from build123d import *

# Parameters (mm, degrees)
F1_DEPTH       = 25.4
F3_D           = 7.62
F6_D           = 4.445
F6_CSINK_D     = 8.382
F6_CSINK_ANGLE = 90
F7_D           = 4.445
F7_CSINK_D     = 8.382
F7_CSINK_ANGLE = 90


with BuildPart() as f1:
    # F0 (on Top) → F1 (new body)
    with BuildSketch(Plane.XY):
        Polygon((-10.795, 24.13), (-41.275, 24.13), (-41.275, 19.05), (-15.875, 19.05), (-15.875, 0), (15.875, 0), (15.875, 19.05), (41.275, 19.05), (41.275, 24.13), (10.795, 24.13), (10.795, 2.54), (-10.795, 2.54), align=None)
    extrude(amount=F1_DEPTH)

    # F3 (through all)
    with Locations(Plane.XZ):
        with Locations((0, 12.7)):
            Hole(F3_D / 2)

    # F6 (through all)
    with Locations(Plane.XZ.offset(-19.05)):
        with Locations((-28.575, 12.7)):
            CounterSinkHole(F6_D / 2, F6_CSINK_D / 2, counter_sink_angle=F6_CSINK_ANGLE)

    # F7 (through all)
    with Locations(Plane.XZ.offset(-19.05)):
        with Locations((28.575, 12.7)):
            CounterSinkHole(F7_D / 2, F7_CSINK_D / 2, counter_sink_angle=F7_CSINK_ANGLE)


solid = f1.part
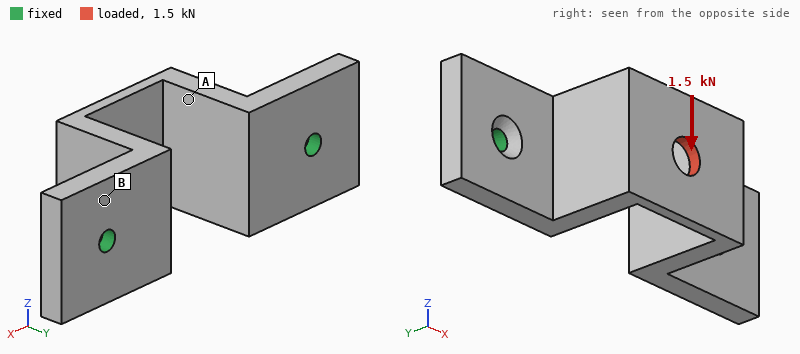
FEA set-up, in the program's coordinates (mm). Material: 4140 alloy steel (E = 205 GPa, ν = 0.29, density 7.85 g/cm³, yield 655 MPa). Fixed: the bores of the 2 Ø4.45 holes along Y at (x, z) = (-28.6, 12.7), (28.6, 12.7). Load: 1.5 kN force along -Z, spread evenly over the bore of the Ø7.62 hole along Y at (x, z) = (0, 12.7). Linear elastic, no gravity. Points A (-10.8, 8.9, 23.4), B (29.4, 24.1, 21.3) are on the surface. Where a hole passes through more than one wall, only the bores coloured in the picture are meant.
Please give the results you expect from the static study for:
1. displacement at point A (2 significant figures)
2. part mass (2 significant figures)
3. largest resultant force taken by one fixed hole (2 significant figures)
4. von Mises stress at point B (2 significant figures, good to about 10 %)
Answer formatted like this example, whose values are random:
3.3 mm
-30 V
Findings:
0.069 mm
110 g
750 N
81 MPa
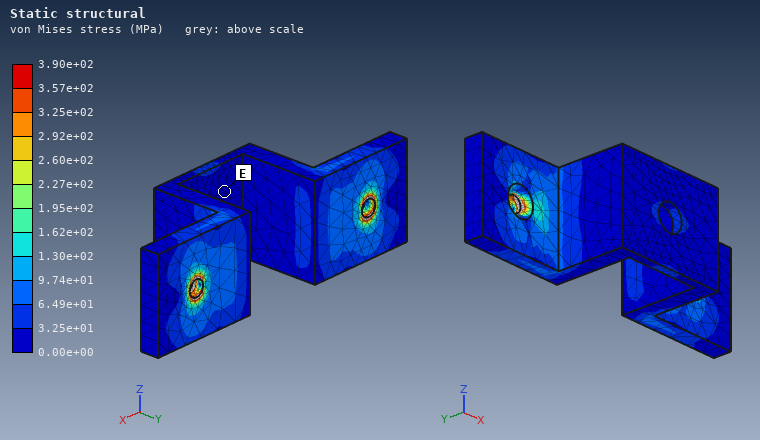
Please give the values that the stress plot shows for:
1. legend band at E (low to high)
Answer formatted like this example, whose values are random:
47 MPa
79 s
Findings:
0.00e+00 to 3.25e+01 MPa
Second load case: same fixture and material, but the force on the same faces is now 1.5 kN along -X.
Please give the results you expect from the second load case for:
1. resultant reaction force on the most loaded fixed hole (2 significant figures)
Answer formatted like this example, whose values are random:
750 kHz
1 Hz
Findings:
880 N
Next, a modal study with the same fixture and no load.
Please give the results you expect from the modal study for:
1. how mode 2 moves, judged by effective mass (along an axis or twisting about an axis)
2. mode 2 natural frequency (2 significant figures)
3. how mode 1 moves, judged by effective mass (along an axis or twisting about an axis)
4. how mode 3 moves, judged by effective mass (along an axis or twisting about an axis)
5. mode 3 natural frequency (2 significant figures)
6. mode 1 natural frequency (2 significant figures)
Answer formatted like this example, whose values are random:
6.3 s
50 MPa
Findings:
along X
4900 Hz
along Z
along Y
6900 Hz
3500 Hz
